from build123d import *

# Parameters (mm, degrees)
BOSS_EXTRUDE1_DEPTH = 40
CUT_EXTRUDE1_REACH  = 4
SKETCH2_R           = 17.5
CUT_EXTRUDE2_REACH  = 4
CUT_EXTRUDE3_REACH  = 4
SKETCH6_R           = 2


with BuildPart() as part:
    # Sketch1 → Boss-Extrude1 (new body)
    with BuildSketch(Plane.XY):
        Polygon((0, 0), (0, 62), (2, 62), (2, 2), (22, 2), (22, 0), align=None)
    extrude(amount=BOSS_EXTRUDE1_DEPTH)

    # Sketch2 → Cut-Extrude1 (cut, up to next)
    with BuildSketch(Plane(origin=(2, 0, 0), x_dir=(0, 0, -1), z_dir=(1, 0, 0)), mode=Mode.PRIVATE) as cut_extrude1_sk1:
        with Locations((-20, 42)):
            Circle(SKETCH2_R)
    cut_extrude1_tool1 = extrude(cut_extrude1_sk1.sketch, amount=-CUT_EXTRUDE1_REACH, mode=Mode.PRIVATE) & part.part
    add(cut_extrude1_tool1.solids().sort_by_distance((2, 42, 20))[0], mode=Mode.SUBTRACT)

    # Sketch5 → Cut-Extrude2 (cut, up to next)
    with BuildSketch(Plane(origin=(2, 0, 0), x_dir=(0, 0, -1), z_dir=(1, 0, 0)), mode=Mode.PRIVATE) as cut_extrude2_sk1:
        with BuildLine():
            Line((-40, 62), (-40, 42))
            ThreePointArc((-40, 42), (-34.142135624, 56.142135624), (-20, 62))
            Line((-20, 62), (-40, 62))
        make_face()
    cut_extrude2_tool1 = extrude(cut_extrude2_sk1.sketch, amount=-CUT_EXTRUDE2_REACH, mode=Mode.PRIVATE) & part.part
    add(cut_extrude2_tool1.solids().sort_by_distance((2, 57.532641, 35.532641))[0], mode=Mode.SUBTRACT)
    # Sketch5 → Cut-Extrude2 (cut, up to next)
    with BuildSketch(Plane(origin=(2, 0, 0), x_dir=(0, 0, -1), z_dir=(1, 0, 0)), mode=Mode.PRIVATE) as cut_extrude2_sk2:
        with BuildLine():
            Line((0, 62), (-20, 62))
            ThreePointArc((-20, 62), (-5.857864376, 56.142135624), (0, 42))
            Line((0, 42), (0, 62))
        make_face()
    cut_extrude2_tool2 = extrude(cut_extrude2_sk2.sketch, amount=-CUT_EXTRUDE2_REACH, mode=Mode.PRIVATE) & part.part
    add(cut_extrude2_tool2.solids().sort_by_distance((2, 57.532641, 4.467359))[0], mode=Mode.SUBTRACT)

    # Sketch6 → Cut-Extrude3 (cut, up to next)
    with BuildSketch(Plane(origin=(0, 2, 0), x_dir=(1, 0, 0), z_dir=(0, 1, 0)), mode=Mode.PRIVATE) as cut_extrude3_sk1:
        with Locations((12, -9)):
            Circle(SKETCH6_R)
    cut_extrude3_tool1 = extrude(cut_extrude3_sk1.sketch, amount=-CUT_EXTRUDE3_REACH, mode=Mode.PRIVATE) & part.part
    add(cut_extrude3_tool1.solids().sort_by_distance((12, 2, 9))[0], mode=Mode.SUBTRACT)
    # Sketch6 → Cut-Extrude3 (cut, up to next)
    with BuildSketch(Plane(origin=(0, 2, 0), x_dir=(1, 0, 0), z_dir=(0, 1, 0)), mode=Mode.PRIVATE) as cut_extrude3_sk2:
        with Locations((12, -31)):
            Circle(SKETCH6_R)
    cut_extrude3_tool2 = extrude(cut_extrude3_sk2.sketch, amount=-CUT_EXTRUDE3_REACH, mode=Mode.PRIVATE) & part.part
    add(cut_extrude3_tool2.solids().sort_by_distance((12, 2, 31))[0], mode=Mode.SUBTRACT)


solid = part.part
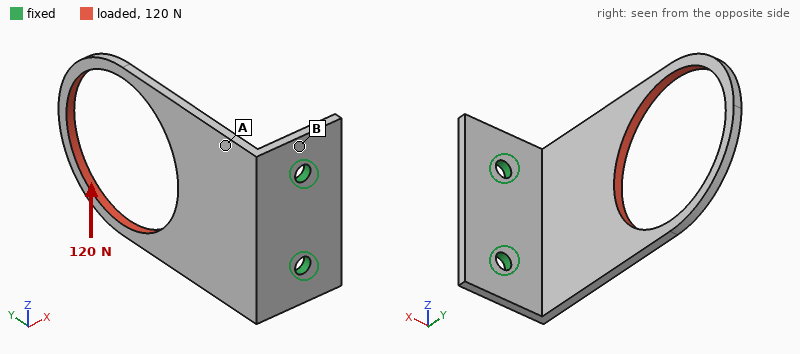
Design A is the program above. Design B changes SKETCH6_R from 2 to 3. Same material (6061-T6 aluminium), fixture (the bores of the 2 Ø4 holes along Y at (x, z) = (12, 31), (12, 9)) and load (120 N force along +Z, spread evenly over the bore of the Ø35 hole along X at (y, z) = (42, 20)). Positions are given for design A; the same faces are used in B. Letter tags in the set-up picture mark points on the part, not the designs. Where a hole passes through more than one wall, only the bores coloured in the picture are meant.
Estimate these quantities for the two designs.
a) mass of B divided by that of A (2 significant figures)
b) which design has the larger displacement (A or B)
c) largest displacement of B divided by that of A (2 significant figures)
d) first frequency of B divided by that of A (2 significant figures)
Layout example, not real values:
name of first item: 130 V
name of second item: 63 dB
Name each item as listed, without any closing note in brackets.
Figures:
mass of B divided by that of A: 0.99
which design has the larger displacement: A
largest displacement of B divided by that of A: 0.85
first frequency of B divided by that of A: 1.0
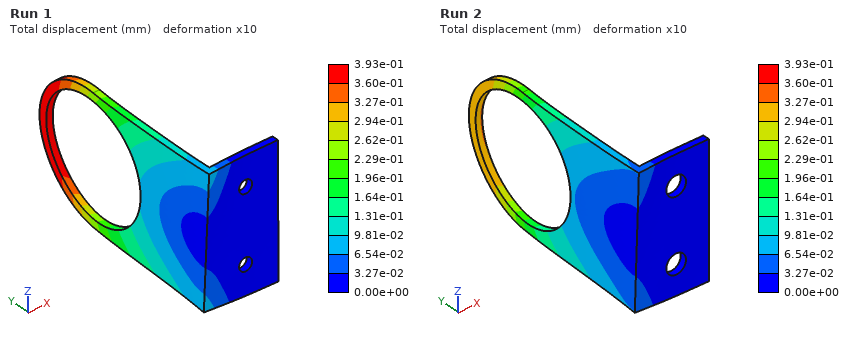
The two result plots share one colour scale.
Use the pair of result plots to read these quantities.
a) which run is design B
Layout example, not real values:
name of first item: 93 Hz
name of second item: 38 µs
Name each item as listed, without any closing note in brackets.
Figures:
which run is design B: Run 2
